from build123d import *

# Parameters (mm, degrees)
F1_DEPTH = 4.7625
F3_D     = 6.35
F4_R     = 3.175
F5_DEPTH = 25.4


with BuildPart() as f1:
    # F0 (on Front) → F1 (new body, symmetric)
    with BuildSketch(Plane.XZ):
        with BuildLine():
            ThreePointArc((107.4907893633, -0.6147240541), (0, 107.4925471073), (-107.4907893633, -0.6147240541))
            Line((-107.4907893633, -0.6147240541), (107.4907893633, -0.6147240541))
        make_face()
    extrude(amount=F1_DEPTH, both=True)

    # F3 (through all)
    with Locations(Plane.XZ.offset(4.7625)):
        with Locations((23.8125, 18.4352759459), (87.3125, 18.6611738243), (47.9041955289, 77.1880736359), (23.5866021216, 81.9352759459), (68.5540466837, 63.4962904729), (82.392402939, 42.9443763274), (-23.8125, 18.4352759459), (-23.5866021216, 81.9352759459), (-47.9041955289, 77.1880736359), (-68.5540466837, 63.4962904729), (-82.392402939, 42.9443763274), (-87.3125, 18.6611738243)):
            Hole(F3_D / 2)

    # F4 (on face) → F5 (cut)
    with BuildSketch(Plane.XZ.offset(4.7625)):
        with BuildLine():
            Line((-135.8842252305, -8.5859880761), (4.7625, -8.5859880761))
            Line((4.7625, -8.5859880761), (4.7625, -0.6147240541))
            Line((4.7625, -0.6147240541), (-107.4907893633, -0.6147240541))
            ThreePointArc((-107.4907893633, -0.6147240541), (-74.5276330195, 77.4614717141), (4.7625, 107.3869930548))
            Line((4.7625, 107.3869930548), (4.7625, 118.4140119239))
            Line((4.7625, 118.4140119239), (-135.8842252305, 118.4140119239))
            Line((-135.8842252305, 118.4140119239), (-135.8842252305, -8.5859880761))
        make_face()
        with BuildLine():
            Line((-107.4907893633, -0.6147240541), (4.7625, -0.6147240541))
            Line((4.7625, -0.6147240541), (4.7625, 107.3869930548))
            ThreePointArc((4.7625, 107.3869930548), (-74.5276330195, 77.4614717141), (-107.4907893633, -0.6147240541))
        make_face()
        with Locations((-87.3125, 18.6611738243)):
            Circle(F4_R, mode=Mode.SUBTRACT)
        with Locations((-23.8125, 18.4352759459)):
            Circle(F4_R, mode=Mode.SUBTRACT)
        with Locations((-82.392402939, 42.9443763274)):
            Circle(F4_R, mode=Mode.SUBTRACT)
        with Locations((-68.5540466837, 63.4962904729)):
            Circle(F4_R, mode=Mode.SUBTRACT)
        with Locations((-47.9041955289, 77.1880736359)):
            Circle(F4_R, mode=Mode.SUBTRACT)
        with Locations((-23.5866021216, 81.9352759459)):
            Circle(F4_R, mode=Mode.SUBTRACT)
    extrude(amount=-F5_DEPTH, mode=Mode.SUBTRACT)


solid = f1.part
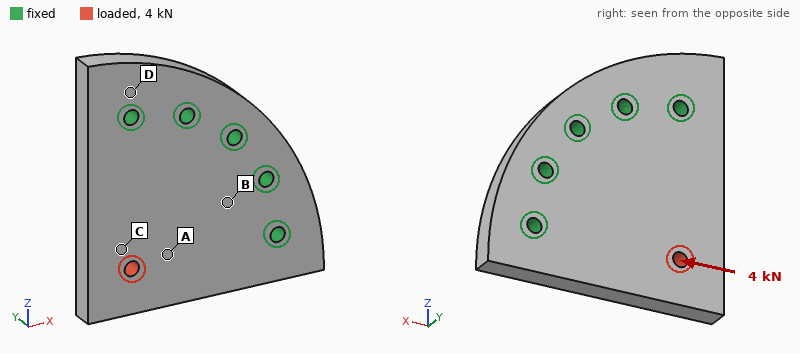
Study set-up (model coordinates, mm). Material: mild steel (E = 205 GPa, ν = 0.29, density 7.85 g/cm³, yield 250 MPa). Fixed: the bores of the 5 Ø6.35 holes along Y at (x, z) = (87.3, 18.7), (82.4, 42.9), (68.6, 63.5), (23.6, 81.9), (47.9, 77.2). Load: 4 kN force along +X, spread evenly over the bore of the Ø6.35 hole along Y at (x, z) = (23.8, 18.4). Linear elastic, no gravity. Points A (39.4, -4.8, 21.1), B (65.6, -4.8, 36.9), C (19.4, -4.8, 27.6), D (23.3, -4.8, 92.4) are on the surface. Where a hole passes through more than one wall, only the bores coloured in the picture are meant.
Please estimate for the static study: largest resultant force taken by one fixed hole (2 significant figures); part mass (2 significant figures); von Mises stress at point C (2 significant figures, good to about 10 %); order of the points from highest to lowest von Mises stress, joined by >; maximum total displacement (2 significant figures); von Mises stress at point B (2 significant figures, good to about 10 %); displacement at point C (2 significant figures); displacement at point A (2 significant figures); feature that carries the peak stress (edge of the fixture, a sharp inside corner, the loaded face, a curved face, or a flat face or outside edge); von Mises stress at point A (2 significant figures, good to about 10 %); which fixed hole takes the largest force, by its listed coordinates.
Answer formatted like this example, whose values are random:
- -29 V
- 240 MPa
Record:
- 2.3 kN
- 630 g
- 9.1 MPa
- A > C > B > D
- 3.9 µm
- 6.5 MPa
- 2.6 µm
- 2.2 µm
- the loaded face
- 13 MPa
- (87.3, 18.7)
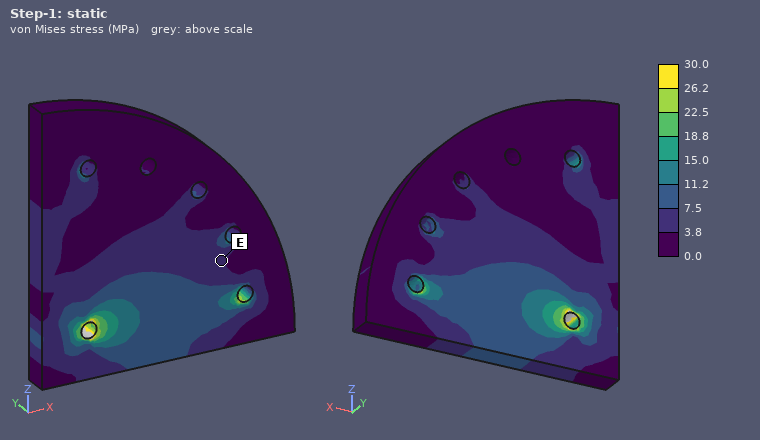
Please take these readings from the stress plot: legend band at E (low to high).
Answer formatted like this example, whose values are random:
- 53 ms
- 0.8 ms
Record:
- 3.8 to 7.5 MPa
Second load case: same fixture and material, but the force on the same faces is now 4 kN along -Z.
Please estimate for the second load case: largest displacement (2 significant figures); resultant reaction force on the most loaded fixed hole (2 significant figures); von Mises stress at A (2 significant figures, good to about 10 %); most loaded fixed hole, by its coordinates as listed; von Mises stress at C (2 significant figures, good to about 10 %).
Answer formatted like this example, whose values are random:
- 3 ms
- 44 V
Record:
- 3.9 µm
- 2.3 kN
- 6.7 MPa
- (23.6, 81.9)
- 15 MPa
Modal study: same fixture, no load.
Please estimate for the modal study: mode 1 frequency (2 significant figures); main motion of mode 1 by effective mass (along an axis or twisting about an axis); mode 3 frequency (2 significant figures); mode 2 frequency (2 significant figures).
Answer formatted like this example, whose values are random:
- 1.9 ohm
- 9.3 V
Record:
- 2200 Hz
- along Y
- 8700 Hz
- 6900 Hz
